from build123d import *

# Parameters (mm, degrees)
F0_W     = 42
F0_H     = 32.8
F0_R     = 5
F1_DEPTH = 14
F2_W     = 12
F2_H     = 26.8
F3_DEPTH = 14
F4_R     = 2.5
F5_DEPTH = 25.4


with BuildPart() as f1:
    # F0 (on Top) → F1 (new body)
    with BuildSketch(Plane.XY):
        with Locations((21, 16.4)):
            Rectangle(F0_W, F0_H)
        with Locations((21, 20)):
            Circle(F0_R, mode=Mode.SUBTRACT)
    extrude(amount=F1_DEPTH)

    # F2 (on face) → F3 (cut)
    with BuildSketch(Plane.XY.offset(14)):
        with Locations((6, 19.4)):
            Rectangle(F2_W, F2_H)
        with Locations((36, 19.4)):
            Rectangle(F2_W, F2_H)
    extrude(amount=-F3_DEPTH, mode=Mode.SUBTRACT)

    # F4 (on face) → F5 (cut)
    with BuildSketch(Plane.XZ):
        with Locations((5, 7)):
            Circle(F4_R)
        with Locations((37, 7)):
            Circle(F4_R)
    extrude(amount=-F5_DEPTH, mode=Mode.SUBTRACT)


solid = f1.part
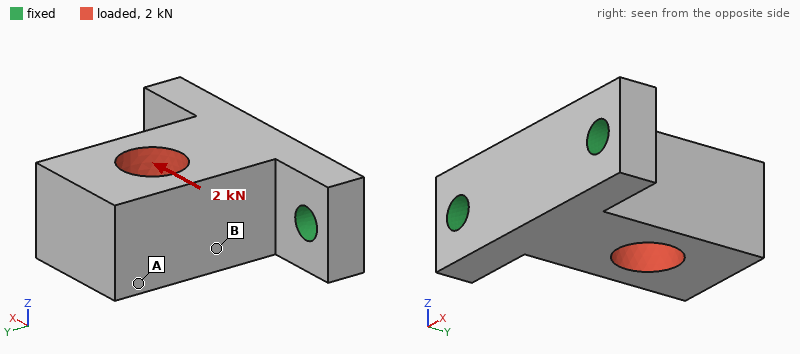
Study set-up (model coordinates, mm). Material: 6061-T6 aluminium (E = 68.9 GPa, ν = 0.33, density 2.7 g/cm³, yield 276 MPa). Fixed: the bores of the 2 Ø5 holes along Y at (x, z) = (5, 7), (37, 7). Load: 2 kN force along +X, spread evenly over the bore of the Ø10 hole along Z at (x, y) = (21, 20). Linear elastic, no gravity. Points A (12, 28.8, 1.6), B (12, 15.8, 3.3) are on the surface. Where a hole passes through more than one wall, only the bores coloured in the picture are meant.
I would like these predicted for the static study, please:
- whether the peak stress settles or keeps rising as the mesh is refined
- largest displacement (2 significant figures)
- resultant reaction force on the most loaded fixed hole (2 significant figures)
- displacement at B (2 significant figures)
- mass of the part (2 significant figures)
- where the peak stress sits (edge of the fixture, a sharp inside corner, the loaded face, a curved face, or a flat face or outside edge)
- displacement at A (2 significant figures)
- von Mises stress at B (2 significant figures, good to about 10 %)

keeps rising
51 µm
1.7 kN
22 µm
24 g
edge of the fixture
46 µm
30 MPa
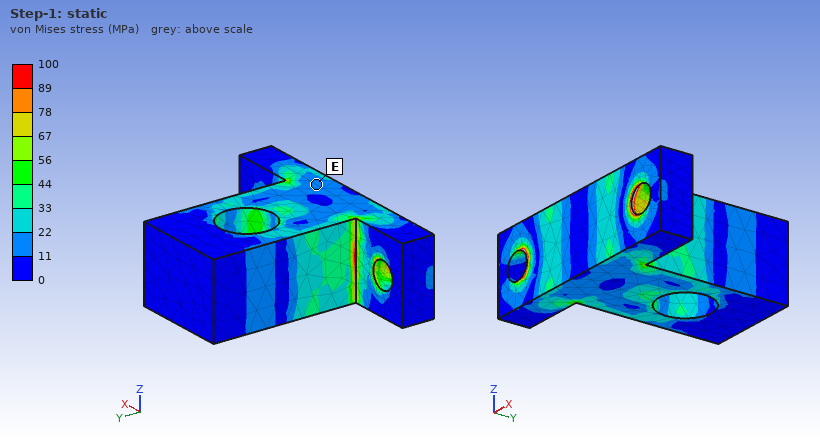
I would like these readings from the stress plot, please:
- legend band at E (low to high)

11 to 22 MPa
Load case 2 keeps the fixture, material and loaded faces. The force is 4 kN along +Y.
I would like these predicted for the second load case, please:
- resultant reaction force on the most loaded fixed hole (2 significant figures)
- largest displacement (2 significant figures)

2.1 kN
22 µm
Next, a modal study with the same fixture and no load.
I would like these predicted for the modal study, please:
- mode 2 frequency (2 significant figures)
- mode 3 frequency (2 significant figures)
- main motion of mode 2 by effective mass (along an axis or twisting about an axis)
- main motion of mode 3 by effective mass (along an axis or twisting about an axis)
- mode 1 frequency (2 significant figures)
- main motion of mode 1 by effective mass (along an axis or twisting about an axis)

9400 Hz
17 kHz
along X
along Y
4800 Hz
along Z
